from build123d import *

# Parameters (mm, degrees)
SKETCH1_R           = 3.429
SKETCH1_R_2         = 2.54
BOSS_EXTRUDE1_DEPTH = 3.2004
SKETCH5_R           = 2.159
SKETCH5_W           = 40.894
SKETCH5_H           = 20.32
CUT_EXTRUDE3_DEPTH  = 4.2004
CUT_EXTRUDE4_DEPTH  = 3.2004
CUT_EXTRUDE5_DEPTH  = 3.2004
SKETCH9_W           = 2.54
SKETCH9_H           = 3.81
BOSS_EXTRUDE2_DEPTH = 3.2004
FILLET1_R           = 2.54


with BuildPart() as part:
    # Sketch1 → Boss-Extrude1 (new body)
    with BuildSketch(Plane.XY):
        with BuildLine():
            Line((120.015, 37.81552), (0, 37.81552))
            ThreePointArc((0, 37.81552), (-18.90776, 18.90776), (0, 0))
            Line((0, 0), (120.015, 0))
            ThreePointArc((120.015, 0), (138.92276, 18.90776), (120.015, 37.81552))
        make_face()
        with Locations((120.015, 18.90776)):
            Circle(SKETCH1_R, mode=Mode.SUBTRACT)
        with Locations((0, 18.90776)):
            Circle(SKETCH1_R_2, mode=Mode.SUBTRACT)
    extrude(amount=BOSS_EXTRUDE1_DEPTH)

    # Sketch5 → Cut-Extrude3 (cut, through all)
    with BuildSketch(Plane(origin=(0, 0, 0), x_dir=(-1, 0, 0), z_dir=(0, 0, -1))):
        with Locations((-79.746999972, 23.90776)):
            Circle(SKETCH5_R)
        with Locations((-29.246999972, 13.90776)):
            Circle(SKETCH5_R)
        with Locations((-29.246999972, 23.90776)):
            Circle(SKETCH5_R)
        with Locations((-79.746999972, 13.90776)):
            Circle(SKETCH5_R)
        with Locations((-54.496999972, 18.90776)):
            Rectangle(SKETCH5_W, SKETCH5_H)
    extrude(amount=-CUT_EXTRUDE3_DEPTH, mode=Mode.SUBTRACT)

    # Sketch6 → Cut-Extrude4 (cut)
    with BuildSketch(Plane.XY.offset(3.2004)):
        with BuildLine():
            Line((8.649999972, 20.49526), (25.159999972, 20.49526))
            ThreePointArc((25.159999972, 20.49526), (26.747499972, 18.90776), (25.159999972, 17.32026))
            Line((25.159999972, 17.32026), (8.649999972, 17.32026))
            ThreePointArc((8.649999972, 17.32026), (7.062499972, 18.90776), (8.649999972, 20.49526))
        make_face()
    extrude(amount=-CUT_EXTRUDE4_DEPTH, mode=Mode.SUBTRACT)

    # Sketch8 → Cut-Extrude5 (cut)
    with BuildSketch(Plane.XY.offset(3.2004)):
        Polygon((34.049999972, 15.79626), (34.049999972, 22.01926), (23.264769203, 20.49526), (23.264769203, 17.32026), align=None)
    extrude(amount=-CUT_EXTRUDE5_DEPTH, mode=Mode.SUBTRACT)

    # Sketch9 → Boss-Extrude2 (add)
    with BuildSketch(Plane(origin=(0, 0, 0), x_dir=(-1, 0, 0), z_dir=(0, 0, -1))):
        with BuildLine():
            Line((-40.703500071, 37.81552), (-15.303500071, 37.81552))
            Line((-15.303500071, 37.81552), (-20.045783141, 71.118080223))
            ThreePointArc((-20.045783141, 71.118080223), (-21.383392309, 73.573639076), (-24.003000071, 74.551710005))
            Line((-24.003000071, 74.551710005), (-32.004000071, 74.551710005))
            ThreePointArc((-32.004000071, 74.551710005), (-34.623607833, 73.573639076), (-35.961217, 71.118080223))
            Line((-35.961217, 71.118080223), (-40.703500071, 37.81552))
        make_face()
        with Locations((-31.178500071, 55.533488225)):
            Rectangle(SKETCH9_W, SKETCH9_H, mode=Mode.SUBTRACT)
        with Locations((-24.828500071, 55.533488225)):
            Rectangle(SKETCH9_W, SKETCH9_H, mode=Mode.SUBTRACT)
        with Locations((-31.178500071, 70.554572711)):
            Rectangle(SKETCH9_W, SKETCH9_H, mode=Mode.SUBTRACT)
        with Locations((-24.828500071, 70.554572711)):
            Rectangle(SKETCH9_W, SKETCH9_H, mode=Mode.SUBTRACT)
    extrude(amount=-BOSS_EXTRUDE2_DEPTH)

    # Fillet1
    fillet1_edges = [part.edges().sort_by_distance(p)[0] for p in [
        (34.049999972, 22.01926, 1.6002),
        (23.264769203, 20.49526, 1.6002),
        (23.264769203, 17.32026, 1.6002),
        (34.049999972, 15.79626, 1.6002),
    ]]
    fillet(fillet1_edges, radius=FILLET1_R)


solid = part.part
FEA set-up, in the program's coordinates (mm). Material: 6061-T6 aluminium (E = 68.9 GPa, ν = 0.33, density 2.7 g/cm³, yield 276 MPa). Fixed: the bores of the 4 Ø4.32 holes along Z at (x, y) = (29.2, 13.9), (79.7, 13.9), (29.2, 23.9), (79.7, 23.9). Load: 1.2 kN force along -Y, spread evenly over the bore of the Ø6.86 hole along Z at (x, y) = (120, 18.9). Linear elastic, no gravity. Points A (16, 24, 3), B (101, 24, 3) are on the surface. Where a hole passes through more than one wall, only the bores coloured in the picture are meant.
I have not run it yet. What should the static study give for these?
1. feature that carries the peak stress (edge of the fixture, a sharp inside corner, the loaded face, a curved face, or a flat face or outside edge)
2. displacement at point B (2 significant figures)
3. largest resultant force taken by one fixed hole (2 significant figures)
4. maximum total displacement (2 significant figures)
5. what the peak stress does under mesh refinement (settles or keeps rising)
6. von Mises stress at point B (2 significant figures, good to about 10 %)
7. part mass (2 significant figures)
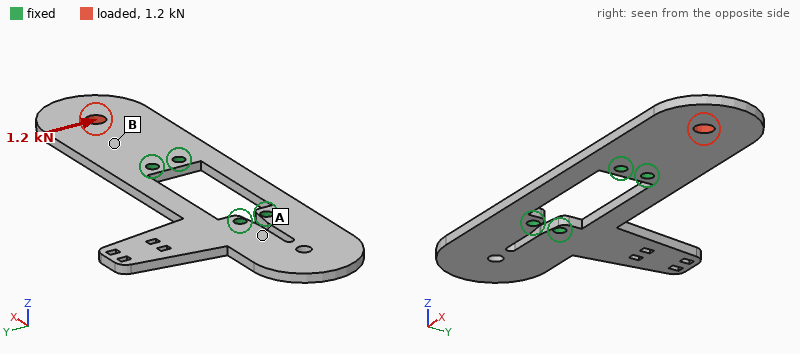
edge of the fixture
0.042 mm
2.3 kN
0.12 mm
keeps rising
27 MPa
46 g
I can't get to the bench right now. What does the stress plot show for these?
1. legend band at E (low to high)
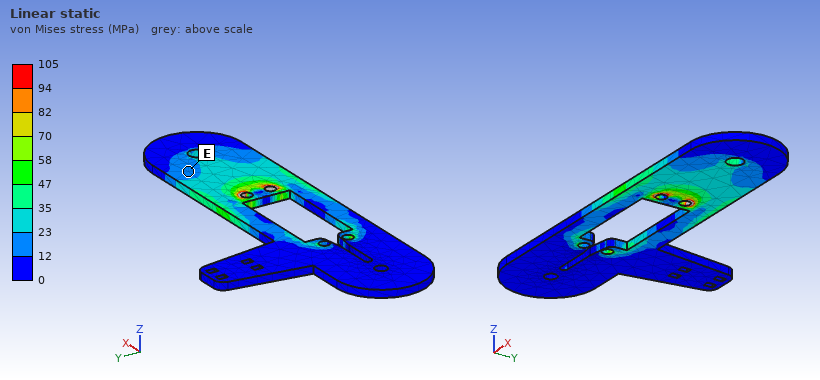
12 to 23 MPa
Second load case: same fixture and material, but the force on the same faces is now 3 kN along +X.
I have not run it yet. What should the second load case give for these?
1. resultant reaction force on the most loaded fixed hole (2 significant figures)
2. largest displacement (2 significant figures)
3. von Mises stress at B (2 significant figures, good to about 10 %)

1.4 kN
24 µm
32 MPa
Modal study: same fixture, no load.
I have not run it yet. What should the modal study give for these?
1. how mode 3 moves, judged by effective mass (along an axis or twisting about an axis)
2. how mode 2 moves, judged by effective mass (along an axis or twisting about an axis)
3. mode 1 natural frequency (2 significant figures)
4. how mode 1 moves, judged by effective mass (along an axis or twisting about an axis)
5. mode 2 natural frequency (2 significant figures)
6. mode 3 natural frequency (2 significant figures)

along Z
twisting about X
880 Hz
along Z
1300 Hz
1300 Hz
